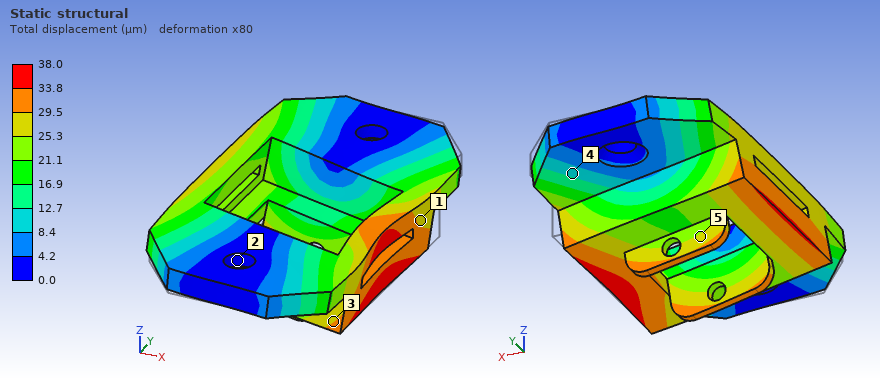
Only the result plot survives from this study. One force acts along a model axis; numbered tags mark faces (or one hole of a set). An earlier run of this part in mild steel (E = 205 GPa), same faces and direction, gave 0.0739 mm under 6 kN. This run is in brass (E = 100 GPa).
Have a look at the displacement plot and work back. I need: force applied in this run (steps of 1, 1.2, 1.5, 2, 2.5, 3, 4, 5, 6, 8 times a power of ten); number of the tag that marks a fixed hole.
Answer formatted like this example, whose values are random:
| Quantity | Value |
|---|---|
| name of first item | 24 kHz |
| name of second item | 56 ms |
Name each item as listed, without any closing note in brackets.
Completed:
| Quantity | Value |
|---|---|
| force applied in this run | 1.5 kN |
| number of the tag that marks a fixed hole | 2 |
